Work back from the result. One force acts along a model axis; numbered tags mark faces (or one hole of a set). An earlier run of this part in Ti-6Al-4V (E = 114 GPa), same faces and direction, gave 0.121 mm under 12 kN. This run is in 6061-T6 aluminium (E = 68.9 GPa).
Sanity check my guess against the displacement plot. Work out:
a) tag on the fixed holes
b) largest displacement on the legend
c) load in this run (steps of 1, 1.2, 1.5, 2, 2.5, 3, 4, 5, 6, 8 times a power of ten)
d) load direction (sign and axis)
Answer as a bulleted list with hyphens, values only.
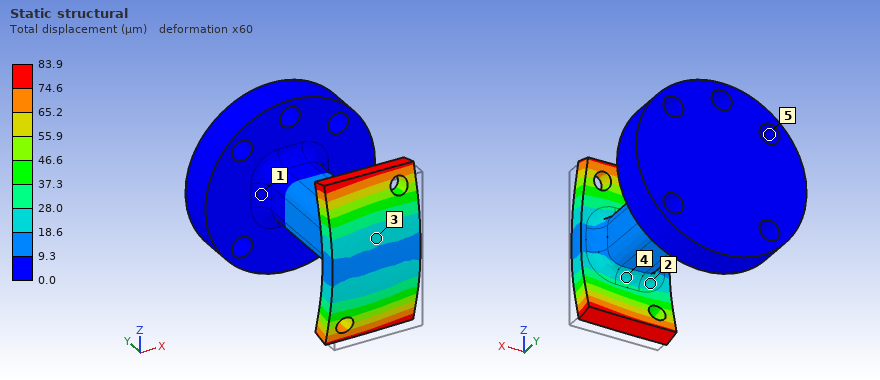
- 5
- 83.9 µm
- 5 kN
- +Y
